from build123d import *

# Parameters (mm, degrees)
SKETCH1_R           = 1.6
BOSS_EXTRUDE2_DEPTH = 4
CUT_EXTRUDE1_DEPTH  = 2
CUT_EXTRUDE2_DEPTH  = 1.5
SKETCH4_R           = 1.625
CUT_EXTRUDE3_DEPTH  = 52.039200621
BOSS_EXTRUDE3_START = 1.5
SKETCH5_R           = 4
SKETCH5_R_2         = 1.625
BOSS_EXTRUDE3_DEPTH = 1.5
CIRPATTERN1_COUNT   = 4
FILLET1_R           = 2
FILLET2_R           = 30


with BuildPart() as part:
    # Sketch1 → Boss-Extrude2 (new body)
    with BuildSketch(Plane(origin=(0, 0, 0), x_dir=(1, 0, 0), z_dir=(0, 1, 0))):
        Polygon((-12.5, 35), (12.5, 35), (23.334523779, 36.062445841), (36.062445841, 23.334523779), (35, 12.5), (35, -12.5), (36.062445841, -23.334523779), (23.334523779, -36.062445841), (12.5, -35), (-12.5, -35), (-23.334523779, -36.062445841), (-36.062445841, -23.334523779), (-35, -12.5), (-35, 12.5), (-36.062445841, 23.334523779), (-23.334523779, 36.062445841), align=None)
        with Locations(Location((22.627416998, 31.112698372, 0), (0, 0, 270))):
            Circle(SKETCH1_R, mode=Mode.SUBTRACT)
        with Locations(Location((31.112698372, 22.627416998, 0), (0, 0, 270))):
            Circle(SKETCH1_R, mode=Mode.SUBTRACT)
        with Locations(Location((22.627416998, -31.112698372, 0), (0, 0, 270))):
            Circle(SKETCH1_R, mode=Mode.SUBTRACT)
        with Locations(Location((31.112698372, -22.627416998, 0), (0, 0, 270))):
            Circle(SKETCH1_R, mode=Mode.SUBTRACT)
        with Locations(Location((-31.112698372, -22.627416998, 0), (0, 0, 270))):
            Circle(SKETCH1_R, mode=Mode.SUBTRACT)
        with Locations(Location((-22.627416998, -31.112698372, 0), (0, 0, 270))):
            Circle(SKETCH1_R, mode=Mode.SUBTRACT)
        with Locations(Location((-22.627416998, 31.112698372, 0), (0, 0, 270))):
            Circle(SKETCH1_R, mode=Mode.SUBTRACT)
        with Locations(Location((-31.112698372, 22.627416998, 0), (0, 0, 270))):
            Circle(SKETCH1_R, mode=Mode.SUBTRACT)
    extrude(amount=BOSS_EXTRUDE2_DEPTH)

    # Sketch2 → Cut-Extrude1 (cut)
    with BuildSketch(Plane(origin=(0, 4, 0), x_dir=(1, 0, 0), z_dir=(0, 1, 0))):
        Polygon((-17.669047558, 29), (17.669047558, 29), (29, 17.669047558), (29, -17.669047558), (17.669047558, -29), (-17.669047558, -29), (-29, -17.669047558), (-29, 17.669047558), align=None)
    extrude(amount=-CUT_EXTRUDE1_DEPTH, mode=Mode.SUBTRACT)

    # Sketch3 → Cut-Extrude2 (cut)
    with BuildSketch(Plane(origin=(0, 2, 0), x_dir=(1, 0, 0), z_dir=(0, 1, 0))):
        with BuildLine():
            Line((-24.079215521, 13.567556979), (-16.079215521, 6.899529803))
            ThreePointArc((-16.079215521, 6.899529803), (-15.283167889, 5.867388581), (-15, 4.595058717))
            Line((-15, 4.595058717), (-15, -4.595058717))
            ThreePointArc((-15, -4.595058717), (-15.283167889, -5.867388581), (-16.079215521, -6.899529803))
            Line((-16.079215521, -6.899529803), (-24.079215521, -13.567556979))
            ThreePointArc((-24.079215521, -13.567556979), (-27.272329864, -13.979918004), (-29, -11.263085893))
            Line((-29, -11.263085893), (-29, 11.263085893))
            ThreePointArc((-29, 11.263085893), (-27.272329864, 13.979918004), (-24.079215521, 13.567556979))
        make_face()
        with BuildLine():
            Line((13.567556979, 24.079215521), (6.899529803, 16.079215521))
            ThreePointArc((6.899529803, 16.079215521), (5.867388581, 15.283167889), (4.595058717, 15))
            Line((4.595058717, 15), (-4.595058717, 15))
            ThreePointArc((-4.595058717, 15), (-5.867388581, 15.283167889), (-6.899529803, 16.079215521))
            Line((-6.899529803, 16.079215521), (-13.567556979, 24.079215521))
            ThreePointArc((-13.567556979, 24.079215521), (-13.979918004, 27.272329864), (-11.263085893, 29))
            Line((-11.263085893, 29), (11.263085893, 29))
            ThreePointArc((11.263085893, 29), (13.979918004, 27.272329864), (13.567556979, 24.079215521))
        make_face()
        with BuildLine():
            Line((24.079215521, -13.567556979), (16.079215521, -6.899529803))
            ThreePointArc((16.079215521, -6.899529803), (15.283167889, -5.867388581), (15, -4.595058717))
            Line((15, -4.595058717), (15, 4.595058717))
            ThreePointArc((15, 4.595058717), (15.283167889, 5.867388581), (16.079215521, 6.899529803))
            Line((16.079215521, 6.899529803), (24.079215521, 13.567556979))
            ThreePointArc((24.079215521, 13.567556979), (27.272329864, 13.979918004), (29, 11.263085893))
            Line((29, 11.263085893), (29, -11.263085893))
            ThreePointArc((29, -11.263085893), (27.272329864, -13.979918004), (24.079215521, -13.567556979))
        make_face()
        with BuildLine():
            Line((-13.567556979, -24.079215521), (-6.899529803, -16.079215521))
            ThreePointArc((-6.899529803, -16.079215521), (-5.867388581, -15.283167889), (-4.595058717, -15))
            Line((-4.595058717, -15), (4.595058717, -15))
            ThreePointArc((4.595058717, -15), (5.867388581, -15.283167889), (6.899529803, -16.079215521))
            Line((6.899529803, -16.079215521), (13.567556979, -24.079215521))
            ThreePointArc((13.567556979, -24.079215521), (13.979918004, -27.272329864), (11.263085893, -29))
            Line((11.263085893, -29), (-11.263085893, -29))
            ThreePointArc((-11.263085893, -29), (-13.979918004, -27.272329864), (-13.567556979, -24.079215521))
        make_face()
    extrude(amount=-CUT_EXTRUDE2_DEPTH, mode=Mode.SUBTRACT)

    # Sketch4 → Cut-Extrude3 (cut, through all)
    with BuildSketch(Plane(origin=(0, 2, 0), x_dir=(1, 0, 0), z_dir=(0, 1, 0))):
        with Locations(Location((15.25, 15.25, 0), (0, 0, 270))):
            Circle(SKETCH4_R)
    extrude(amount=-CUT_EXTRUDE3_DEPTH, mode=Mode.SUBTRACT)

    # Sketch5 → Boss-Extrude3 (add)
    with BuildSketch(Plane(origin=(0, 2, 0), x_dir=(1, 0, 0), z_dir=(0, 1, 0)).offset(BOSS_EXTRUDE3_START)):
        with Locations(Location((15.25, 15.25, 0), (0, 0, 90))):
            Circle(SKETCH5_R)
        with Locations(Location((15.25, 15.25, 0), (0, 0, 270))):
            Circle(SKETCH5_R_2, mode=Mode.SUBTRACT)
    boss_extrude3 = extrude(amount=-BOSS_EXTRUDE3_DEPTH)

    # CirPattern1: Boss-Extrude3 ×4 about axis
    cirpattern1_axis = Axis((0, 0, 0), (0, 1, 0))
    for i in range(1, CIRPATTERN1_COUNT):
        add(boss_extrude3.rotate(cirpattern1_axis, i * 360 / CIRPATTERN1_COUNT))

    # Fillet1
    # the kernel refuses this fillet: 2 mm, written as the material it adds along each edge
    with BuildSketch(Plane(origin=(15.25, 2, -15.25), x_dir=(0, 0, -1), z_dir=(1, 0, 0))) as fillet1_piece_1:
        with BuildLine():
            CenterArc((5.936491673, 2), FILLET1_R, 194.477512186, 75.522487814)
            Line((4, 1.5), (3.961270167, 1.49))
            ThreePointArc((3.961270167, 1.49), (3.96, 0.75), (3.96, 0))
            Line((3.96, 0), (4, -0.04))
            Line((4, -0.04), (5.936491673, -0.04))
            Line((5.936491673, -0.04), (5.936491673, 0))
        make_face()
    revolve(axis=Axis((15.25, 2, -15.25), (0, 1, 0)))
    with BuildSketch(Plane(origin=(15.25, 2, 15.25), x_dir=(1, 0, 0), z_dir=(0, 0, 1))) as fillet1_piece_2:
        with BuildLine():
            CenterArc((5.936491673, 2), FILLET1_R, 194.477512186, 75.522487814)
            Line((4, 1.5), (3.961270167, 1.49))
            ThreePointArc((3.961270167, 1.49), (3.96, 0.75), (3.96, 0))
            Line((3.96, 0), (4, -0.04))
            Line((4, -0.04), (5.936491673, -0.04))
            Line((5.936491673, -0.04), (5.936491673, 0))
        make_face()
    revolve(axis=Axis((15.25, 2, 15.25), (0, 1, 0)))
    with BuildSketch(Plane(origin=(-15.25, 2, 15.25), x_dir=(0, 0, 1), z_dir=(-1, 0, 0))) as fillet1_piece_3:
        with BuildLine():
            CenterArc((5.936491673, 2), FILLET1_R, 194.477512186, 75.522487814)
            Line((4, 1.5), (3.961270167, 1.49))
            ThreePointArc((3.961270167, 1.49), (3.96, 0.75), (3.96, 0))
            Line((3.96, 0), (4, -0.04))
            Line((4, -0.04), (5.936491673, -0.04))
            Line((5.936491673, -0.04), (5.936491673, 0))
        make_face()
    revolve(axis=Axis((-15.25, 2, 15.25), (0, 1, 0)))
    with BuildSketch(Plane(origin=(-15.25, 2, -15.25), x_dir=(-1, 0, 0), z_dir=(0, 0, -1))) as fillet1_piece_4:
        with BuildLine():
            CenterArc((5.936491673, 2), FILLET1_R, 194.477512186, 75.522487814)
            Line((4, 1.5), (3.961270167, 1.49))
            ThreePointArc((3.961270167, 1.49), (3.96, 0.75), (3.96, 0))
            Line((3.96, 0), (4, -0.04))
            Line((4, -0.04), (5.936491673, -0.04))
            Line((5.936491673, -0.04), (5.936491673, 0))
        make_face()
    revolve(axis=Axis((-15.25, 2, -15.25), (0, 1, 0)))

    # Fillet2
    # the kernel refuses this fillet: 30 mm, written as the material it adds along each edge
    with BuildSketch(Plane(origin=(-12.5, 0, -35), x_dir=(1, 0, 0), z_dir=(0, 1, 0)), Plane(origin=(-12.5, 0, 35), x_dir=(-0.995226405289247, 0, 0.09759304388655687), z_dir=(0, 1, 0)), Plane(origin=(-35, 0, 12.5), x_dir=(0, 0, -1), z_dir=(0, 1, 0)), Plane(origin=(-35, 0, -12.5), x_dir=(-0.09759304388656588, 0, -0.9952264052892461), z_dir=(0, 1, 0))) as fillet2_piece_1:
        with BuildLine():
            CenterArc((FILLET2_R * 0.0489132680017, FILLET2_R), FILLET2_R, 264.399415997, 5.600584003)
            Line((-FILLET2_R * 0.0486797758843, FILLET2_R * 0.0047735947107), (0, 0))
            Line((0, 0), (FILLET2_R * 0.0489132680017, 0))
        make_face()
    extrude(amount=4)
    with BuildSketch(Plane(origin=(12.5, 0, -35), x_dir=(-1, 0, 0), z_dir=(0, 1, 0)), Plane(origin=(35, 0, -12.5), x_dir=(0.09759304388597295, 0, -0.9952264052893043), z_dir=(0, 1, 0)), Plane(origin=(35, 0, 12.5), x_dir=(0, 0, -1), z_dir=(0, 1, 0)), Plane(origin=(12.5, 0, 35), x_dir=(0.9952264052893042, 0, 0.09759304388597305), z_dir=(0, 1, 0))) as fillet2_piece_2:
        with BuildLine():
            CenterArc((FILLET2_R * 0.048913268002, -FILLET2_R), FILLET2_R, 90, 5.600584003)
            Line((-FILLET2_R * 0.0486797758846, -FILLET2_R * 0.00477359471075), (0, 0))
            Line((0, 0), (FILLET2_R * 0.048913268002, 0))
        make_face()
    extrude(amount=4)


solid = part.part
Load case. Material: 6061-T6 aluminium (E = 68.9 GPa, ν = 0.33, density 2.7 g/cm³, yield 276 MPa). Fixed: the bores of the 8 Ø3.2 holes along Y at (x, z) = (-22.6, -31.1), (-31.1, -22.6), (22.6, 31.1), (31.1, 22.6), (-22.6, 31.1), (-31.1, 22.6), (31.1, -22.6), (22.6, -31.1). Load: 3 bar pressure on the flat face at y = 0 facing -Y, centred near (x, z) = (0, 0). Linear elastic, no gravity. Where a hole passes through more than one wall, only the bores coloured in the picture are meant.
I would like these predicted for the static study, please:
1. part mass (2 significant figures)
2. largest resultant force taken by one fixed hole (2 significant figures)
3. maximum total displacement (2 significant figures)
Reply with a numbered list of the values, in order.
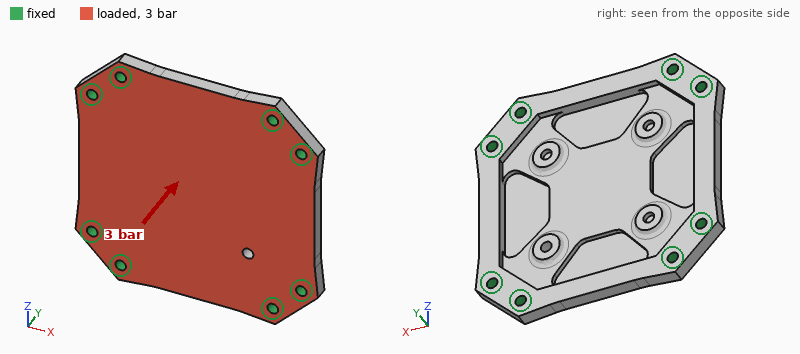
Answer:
1. 29 g
2. 220 N
3. 0.22 mm
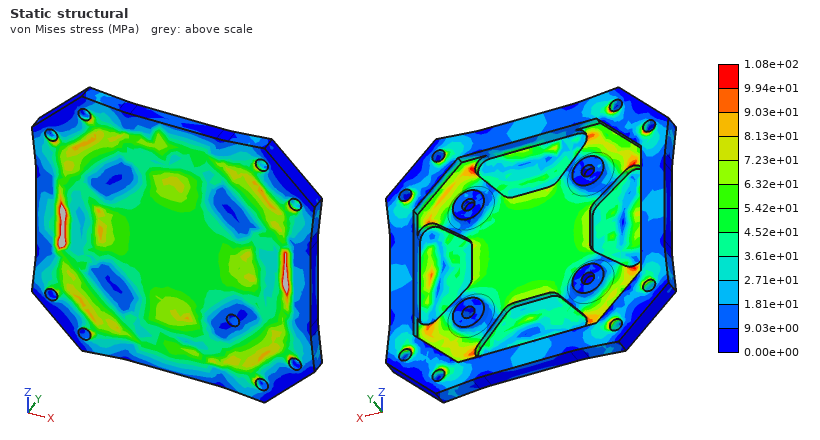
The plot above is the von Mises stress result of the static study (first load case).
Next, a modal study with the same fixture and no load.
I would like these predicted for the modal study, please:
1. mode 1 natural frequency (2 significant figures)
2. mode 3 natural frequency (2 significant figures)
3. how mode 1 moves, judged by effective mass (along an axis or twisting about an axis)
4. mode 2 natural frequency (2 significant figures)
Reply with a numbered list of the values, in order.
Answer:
1. 3300 Hz
2. 7200 Hz
3. along Y
4. 7100 Hz
